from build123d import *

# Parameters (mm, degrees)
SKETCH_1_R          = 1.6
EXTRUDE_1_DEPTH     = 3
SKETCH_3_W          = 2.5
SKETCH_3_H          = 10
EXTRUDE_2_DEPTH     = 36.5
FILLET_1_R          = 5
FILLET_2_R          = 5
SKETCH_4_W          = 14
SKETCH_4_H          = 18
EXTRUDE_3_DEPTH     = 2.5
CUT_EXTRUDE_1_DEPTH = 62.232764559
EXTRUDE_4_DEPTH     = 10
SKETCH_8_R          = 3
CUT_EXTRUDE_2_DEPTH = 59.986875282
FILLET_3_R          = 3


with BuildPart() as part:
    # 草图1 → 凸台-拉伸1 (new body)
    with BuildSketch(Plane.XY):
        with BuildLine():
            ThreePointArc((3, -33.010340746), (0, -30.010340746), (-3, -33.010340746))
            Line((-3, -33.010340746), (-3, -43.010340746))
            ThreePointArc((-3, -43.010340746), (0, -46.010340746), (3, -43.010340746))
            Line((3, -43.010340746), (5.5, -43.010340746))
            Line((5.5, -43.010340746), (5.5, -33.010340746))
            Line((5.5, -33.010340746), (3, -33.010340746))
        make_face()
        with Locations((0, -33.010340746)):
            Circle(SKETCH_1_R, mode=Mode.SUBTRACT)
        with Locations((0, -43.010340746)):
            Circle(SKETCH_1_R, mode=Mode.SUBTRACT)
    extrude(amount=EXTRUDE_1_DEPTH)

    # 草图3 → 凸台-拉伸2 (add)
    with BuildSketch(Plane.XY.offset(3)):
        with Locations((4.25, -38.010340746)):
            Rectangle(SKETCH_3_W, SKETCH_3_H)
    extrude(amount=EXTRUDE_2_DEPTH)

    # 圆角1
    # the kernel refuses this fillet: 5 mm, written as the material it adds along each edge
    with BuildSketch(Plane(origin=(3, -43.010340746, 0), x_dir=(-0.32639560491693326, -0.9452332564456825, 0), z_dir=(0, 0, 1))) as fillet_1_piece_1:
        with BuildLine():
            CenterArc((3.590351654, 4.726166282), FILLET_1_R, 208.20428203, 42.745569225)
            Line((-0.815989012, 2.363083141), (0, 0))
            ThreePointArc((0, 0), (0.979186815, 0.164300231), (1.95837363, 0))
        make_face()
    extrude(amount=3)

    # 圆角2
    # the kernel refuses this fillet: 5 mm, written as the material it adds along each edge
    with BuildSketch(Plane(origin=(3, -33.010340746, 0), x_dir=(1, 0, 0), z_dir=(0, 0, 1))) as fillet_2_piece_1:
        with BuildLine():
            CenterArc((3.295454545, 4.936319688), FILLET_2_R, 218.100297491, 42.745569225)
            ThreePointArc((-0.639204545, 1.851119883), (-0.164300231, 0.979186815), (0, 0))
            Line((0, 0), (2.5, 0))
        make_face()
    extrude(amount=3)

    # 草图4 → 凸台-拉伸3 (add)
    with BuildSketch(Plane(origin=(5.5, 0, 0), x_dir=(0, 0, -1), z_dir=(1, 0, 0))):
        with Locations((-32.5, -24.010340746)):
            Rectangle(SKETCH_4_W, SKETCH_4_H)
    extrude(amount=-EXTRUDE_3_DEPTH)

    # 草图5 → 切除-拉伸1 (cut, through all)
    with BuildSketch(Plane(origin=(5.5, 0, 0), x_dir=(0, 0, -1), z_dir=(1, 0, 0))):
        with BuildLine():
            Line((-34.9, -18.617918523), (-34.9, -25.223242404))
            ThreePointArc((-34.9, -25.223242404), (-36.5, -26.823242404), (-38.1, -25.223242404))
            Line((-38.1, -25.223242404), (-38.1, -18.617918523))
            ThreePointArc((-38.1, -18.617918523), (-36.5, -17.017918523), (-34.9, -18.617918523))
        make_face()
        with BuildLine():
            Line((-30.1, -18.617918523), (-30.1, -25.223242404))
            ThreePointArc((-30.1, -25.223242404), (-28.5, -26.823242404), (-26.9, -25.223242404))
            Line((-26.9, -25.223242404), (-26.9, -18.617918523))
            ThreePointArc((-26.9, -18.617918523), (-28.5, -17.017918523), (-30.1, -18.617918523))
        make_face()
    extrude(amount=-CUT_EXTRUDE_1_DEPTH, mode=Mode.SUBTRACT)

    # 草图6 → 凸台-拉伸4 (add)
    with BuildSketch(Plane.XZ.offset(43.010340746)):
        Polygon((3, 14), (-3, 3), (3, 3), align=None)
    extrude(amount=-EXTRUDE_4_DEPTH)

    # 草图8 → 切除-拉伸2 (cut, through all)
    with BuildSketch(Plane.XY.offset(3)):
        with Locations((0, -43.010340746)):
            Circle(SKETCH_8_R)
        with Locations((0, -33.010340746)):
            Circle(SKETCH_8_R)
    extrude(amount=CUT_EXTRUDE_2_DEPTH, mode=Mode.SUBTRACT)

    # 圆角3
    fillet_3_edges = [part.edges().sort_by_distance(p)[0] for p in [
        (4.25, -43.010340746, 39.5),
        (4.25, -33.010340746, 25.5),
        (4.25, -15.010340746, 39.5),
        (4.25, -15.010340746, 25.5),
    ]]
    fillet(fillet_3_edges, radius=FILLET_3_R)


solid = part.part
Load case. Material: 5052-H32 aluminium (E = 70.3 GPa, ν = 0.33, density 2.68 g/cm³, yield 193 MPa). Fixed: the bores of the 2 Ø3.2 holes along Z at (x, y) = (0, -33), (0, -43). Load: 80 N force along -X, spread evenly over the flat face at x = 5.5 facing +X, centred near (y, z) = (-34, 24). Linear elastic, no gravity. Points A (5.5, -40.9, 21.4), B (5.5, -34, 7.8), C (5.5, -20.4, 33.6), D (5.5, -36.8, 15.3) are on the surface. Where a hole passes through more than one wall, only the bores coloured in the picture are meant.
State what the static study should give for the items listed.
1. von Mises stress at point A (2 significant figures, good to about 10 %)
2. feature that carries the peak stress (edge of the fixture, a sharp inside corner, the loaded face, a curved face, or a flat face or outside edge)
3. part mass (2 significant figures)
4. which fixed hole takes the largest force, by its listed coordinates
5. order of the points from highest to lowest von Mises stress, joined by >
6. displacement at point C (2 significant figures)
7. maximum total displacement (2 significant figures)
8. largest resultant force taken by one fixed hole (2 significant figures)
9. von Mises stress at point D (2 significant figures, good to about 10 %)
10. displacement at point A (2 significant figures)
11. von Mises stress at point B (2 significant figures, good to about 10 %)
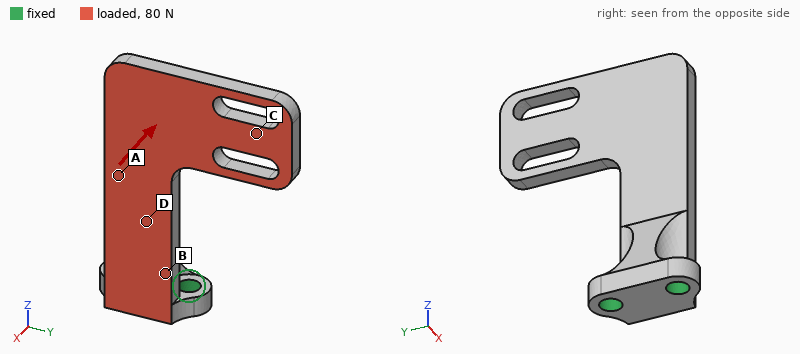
54 MPa
a flat face or outside edge
5.0 g
(0, -33)
D > A > B > C
0.34 mm
0.44 mm
74 N
78 MPa
0.076 mm
37 MPa
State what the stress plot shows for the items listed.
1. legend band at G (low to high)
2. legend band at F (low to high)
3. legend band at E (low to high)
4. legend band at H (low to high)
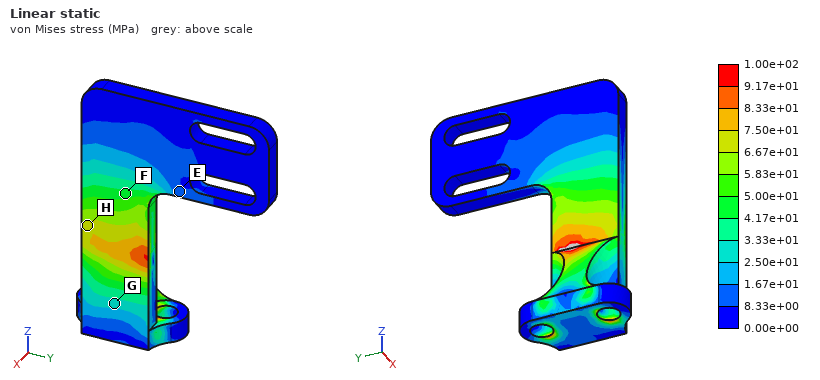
2.50e+01 to 3.33e+01 MPa
4.17e+01 to 5.00e+01 MPa
8.33e+00 to 1.67e+01 MPa
6.67e+01 to 7.50e+01 MPa
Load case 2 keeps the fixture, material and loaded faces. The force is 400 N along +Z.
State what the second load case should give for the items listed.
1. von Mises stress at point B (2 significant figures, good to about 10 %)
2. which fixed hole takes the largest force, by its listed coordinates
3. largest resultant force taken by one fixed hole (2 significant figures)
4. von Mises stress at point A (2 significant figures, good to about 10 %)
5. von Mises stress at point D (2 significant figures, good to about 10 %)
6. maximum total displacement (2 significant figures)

57 MPa
(0, -33)
400 N
16 MPa
54 MPa
0.25 mm
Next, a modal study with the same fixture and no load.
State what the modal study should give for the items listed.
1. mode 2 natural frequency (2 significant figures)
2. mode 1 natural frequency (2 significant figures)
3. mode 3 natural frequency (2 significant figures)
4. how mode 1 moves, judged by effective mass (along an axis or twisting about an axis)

3200 Hz
1400 Hz
3400 Hz
along X
